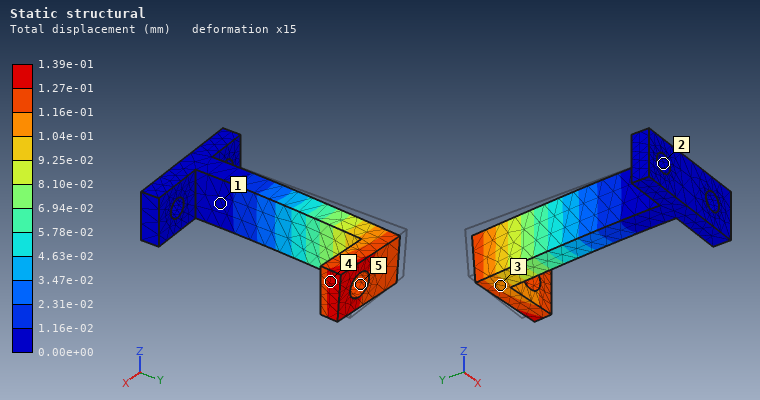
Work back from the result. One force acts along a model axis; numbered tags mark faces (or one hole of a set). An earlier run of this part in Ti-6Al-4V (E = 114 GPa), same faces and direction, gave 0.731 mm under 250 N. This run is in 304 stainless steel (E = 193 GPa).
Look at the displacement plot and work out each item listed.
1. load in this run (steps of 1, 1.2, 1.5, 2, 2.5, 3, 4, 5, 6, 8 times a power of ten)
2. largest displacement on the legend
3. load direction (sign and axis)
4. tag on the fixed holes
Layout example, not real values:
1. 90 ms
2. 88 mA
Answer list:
1. 80 N
2. 1.39e-01 mm
3. +X
4. 2
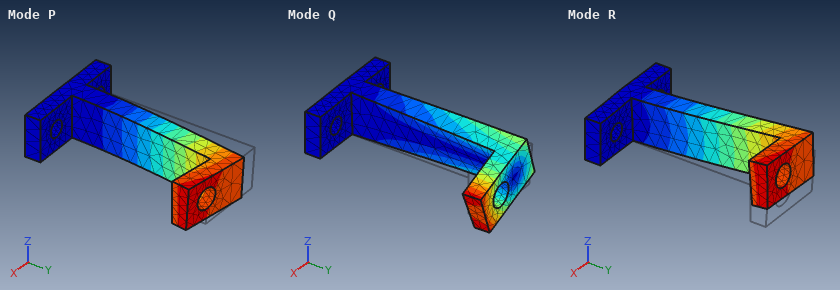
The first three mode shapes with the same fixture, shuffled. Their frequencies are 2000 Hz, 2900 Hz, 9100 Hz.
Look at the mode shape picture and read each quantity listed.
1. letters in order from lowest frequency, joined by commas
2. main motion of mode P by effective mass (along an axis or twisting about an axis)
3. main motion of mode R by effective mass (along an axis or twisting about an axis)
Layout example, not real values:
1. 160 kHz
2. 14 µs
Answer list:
1. P, R, Q
2. along X
3. along Z
